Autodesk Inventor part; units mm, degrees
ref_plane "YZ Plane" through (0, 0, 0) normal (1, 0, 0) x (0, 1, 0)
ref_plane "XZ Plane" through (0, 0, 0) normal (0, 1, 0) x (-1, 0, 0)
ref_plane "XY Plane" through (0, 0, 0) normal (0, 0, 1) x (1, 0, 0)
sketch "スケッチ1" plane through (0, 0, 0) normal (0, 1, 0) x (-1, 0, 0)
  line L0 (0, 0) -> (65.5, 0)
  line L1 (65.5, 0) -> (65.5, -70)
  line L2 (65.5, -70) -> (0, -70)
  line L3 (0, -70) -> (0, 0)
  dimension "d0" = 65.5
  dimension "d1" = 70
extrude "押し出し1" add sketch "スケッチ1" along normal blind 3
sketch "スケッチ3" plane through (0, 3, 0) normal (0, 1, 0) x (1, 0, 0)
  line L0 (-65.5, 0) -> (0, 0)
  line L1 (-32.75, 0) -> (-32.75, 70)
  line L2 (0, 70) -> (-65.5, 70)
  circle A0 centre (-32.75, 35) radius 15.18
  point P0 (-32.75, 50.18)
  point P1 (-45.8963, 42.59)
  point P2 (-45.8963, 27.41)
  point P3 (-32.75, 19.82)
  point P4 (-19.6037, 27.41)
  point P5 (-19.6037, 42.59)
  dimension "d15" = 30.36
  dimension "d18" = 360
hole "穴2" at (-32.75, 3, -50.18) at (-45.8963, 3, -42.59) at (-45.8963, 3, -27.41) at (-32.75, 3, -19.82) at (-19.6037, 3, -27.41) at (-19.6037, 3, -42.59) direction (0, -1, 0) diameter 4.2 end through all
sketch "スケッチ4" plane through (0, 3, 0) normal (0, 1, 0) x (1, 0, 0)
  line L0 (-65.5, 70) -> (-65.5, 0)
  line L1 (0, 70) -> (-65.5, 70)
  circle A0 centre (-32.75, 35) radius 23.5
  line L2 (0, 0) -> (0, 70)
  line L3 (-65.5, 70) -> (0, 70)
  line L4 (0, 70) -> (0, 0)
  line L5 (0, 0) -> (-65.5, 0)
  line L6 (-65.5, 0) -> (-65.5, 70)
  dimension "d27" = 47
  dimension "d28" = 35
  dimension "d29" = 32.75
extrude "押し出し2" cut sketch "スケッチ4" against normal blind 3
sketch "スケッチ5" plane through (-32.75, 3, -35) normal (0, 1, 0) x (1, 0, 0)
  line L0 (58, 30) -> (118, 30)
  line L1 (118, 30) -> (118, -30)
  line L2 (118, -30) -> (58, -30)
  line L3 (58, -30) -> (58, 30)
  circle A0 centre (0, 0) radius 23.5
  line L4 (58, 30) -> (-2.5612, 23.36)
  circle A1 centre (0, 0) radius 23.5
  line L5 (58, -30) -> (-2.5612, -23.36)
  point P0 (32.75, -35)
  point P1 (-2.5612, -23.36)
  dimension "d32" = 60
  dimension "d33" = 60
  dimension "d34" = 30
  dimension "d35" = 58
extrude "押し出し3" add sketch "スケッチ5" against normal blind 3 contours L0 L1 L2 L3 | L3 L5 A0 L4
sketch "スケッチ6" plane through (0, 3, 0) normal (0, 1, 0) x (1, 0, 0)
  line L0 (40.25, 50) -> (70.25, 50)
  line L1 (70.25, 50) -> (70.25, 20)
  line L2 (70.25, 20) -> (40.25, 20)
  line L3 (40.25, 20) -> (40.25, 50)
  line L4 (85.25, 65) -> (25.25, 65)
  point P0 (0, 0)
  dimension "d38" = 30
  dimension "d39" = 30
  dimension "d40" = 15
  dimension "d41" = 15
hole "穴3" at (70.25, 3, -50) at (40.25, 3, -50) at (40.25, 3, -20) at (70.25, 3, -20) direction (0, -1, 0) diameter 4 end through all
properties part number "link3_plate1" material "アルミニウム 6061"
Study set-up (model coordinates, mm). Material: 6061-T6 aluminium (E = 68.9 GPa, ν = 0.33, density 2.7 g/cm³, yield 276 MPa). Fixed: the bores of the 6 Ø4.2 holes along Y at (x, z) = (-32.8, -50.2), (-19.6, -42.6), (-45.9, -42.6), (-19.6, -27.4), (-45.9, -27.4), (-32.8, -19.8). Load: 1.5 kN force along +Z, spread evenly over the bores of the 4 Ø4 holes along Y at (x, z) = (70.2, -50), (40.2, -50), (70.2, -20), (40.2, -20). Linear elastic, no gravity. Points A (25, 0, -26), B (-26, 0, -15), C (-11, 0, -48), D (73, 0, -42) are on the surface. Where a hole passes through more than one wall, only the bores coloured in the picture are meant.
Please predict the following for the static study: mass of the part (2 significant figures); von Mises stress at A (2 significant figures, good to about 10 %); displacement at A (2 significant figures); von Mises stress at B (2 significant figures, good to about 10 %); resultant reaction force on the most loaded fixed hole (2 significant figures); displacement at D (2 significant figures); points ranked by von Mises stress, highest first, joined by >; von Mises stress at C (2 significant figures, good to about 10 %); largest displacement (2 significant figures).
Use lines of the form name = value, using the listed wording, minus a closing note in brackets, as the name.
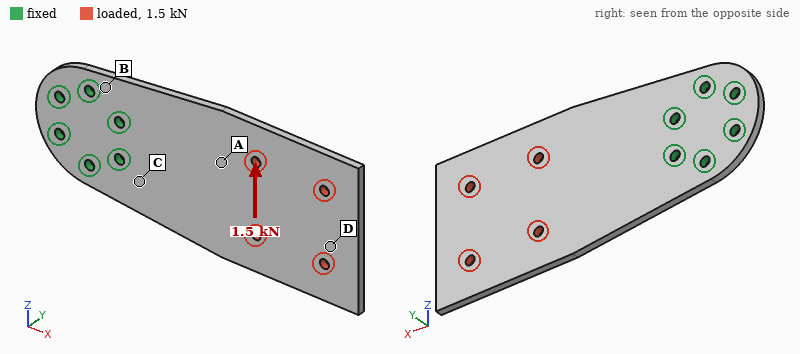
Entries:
mass of the part = 60 g
von Mises stress at A = 23 MPa
displacement at A = 0.087 mm
von Mises stress at B = 64 MPa
resultant reaction force on the most loaded fixed hole = 2.3 kN
displacement at D = 0.20 mm
points ranked by von Mises stress, highest first, joined by > = B > C > A > D
von Mises stress at C = 44 MPa
largest displacement = 0.24 mm
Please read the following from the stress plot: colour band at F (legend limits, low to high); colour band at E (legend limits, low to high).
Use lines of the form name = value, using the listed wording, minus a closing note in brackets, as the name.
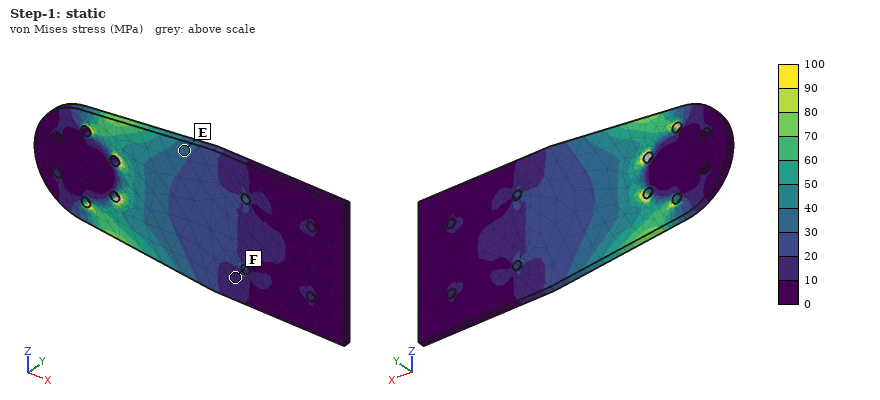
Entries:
colour band at F = 10 to 20 MPa
colour band at E = 30 to 40 MPa
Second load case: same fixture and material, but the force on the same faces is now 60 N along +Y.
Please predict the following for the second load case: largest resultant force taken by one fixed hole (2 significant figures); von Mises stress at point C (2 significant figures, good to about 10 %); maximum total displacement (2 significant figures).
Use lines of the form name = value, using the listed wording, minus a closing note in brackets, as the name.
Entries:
largest resultant force taken by one fixed hole = 98 N
von Mises stress at point C = 47 MPa
maximum total displacement = 1.5 mm
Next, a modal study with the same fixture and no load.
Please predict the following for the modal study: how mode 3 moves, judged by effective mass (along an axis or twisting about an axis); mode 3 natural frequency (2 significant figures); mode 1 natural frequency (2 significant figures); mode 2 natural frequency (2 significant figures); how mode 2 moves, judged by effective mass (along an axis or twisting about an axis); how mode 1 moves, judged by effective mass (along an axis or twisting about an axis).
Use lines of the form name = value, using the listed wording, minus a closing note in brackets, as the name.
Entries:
how mode 3 moves, judged by effective mass = along Y
mode 3 natural frequency = 1400 Hz
mode 1 natural frequency = 220 Hz
mode 2 natural frequency = 770 Hz
how mode 2 moves, judged by effective mass = twisting about X
how mode 1 moves, judged by effective mass = along Y
